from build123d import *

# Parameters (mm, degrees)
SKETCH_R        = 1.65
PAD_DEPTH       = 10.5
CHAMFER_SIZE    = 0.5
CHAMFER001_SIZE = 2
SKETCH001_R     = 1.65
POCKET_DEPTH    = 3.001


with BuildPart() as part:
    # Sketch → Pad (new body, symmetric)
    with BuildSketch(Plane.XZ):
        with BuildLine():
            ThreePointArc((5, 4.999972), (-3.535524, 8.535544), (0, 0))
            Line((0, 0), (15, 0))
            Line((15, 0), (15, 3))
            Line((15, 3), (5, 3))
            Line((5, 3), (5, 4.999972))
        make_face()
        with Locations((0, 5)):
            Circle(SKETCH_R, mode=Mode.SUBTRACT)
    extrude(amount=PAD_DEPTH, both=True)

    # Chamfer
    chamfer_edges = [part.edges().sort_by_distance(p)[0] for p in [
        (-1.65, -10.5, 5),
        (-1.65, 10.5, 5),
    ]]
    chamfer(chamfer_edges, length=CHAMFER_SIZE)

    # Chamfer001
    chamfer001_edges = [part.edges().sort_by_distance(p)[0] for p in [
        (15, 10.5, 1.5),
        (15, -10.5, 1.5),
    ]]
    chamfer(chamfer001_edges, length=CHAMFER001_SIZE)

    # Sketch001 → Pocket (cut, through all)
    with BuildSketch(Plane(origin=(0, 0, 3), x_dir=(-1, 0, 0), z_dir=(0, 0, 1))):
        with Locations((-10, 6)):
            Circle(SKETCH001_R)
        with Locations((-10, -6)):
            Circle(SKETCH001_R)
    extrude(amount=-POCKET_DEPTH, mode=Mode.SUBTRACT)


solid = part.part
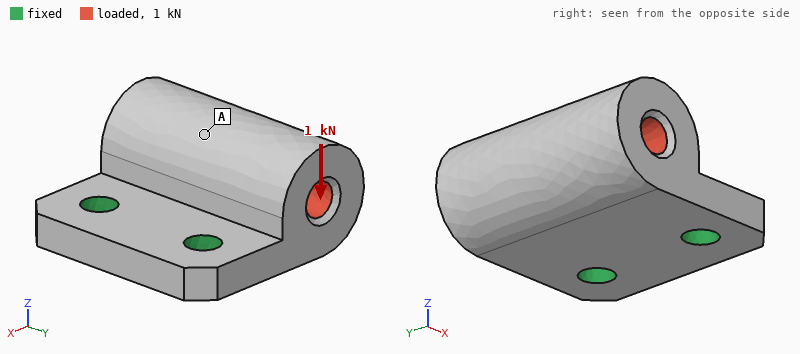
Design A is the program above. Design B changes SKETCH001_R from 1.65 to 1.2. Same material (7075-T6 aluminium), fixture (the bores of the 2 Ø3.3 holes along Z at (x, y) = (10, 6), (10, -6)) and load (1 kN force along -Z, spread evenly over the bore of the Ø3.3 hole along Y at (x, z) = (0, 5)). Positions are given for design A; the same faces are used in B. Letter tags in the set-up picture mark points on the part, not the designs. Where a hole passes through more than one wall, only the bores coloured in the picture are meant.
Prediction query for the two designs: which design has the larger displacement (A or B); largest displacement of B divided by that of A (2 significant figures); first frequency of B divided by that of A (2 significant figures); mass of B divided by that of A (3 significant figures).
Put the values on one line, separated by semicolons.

B; 1.2; 0.91; 1.01
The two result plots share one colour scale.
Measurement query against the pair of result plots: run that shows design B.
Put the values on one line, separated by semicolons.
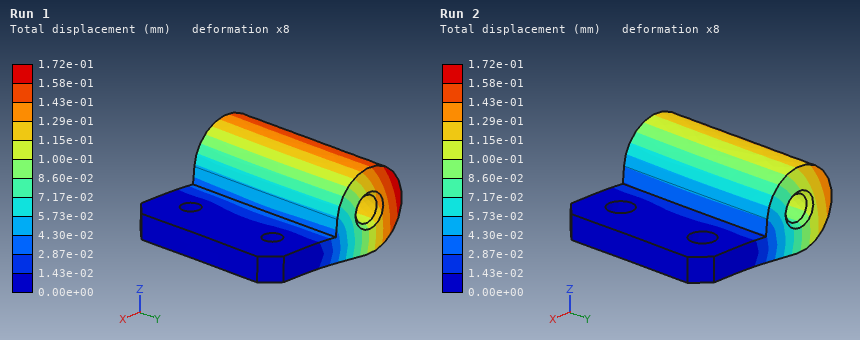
Run 1
